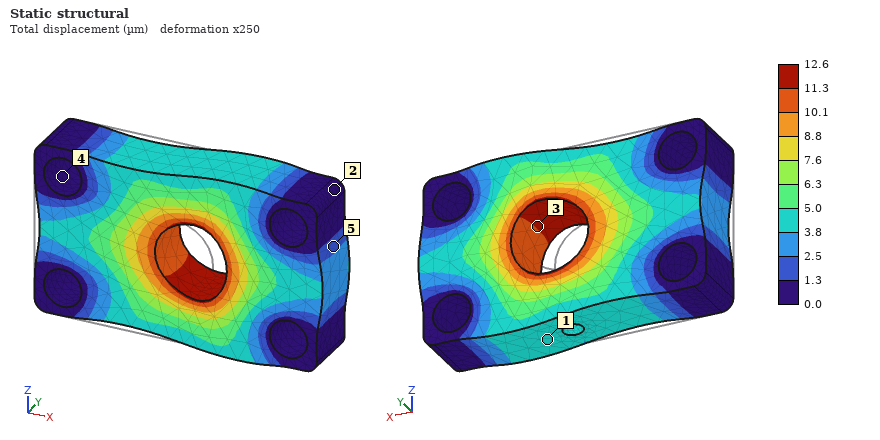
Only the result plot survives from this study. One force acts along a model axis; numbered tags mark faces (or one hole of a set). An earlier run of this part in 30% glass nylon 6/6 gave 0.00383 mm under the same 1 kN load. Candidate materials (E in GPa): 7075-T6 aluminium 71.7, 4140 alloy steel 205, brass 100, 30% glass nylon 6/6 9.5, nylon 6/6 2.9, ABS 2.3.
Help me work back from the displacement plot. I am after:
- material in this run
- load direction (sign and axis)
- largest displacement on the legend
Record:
nylon 6/6
+X
12.6 µm
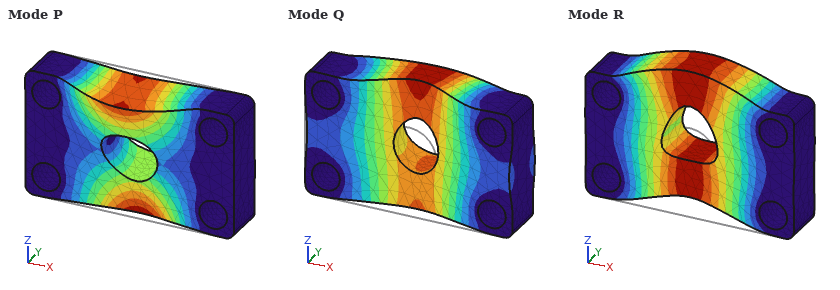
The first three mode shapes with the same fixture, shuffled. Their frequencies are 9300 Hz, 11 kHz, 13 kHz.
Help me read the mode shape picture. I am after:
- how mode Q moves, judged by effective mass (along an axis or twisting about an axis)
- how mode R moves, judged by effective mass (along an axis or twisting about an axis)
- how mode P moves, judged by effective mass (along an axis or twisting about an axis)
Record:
along Y
along Z
twisting about X
